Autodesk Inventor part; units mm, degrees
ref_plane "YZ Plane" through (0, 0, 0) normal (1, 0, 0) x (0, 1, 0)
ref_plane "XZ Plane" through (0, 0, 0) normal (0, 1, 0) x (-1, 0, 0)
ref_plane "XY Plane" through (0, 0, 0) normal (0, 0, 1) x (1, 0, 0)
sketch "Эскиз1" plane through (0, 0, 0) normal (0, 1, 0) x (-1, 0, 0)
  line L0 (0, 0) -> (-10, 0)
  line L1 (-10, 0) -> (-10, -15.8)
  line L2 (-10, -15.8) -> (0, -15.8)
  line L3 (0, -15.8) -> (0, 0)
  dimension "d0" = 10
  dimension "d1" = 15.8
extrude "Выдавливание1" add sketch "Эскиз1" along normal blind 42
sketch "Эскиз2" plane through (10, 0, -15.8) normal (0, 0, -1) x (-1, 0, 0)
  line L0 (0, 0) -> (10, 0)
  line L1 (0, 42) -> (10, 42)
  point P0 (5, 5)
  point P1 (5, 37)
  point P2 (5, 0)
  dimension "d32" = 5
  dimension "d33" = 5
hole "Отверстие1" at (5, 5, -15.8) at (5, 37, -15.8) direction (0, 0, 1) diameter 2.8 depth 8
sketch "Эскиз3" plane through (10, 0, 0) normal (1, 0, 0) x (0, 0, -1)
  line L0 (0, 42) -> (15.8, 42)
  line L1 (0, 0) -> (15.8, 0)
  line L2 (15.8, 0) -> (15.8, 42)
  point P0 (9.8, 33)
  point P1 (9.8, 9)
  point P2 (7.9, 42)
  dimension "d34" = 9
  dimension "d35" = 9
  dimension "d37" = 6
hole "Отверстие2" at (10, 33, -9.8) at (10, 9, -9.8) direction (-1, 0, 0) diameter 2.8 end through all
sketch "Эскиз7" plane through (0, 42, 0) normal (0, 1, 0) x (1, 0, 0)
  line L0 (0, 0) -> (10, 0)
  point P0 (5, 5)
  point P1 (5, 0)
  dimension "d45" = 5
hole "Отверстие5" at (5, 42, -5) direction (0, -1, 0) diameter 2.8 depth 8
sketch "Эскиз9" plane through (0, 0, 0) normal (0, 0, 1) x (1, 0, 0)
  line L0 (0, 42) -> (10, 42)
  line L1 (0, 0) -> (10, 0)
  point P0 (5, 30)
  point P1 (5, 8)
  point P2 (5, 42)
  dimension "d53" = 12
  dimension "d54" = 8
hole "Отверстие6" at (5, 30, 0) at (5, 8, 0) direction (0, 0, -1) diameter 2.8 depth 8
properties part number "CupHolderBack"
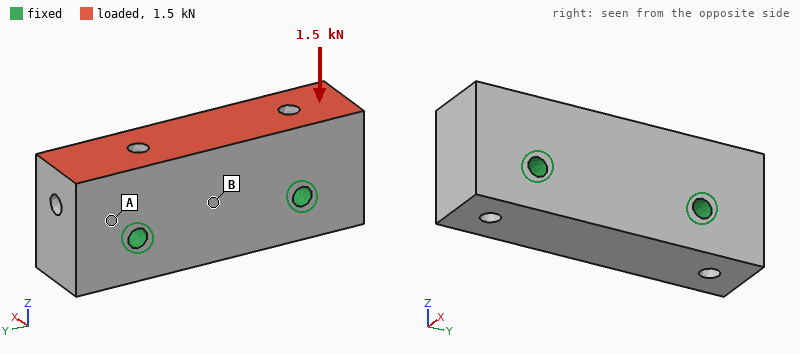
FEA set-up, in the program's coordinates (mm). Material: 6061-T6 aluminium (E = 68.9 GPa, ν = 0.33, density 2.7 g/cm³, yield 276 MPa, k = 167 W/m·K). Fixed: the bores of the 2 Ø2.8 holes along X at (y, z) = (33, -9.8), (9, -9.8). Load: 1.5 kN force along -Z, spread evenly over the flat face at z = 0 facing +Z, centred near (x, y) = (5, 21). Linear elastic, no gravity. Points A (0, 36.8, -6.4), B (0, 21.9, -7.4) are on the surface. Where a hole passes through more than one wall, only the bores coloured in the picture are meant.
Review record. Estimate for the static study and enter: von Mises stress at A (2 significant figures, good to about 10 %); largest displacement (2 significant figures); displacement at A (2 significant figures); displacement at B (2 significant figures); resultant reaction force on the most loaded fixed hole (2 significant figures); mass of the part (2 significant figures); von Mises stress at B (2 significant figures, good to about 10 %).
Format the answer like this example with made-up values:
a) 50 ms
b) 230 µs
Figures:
a) 4.4 MPa
b) 1.5 µm
c) 0.66 µm
d) 0.98 µm
e) 760 N
f) 17 g
g) 1.6 MPa
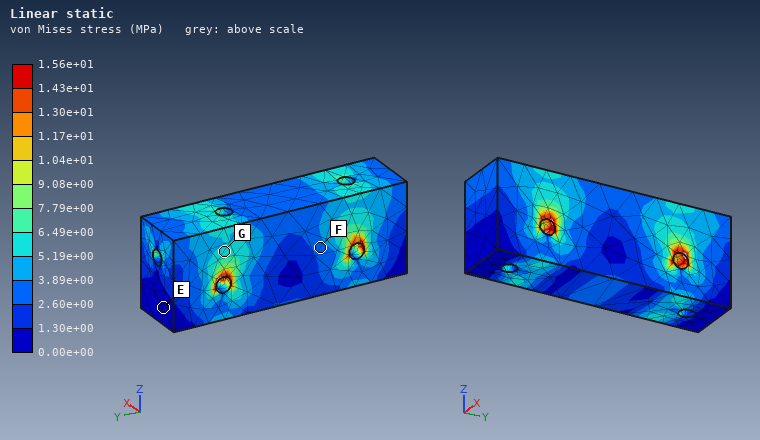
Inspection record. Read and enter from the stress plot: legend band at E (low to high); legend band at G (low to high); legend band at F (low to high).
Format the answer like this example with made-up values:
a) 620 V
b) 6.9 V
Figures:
a) 0.00e+00 to 1.30e+00 MPa
b) 5.19e+00 to 6.49e+00 MPa
c) 2.60e+00 to 3.89e+00 MPa
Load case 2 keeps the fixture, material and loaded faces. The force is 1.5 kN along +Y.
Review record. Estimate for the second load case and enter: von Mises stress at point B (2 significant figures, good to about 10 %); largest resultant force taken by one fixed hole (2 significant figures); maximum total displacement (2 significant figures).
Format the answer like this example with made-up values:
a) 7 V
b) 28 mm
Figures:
a) 8.0 MPa
b) 930 N
c) 4.9 µm
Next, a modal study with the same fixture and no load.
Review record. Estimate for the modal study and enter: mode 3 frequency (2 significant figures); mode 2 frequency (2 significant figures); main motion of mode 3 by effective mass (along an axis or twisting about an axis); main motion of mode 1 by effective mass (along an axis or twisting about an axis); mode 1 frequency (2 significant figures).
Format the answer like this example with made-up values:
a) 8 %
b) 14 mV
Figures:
a) 42 kHz
b) 39 kHz
c) twisting about Z
d) along X
e) 34 kHz
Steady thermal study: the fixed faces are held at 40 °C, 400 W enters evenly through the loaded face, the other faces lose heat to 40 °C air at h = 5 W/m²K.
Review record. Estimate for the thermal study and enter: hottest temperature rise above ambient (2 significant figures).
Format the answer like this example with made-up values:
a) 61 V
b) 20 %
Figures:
a) 83 K
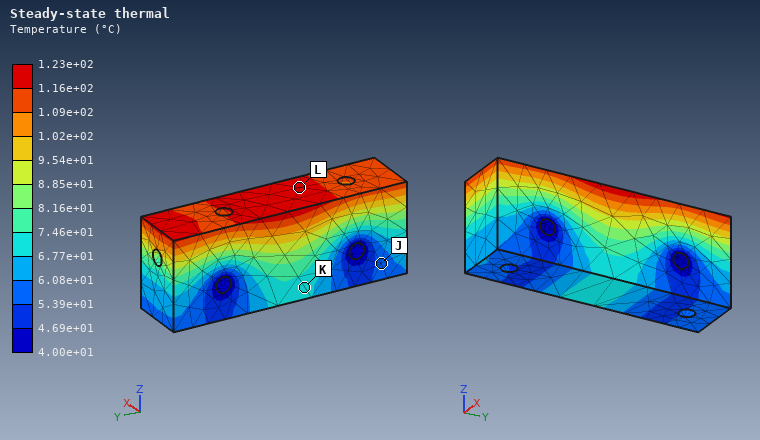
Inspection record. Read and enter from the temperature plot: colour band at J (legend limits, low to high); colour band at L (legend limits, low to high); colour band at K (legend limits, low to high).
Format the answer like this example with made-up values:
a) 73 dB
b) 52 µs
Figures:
a) 5.39e+01 to 6.08e+01 °C
b) 1.16e+02 to 1.23e+02 °C
c) 6.77e+01 to 7.46e+01 °C
